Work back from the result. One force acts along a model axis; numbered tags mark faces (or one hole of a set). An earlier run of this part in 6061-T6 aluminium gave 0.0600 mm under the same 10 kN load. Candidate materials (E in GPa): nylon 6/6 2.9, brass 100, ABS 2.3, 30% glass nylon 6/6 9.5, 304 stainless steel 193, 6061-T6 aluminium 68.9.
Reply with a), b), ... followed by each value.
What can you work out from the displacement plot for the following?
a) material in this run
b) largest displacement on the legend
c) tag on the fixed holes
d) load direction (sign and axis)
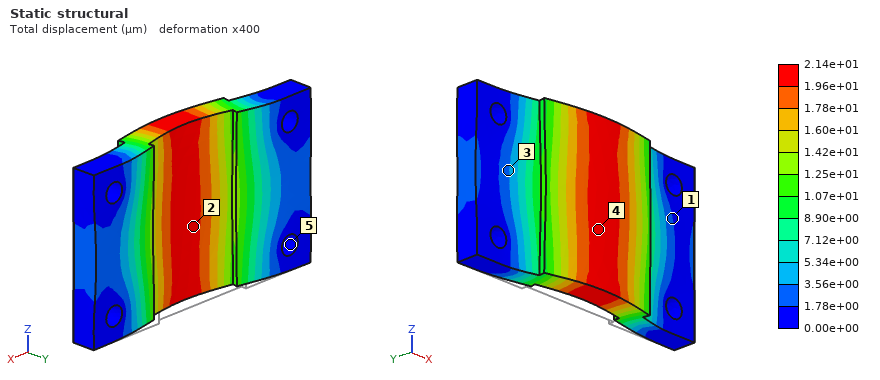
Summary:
a) 304 stainless steel
b) 2.14e+01 µm
c) 5
d) -Y
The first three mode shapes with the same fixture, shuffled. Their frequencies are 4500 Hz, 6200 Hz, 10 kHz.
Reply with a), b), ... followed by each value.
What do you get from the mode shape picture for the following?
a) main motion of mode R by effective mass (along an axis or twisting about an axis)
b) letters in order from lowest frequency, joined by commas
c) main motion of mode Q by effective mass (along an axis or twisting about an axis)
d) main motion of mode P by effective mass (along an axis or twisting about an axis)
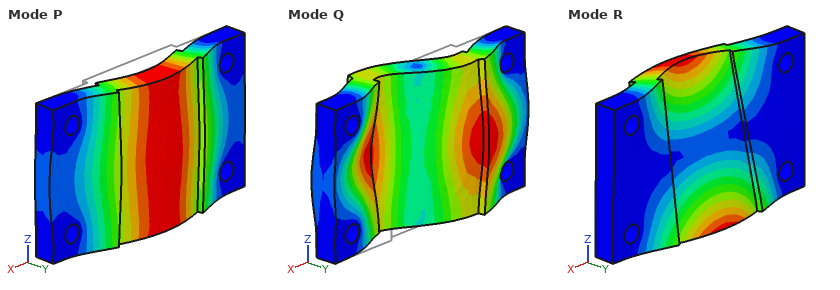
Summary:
a) twisting about X
b) P, R, Q
c) twisting about Z
d) along Y
